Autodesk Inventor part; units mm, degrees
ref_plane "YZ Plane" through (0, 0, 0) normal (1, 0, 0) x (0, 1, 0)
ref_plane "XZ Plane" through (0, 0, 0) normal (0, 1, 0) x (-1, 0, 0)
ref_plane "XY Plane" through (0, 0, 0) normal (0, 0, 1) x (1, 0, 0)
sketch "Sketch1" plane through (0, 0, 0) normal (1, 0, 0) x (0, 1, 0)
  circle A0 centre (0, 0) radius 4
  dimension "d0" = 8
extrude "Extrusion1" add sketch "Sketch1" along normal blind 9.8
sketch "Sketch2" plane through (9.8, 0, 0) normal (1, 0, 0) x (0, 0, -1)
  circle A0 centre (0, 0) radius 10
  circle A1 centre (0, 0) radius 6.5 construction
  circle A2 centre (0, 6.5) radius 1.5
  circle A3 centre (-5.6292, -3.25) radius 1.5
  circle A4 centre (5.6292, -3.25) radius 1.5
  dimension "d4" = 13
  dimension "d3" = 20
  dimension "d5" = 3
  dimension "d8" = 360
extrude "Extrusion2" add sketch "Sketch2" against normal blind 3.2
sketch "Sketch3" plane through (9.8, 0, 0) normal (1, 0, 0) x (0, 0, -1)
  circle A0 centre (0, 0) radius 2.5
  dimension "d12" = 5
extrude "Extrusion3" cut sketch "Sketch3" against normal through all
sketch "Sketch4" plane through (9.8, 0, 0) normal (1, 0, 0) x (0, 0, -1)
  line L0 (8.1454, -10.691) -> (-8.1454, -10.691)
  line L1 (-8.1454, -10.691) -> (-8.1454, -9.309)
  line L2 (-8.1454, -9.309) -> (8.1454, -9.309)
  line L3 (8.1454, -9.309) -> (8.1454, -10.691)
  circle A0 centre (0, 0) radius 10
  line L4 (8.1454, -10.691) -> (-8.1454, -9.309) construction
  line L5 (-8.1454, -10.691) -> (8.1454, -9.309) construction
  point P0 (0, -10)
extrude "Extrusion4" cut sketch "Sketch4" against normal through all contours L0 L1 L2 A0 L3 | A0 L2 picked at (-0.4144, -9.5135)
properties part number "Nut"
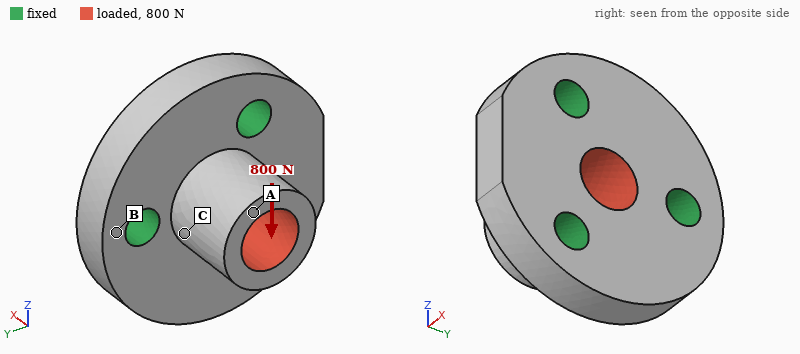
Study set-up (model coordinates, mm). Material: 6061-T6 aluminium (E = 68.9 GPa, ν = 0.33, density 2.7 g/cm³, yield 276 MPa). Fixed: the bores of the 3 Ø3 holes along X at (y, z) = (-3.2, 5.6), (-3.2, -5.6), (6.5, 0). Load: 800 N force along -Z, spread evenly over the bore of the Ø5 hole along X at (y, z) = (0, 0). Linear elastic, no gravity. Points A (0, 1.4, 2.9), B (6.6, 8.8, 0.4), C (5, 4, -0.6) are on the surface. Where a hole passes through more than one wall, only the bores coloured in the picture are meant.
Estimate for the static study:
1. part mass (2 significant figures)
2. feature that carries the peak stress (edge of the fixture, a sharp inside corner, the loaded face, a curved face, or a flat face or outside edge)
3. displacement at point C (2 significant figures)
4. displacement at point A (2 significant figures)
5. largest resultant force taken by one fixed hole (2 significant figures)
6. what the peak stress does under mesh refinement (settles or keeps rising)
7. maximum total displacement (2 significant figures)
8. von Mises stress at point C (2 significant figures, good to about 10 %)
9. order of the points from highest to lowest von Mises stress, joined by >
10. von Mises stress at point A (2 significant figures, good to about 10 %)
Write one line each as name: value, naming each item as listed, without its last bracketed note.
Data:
part mass: 2.9 g
feature that carries the peak stress: a sharp inside corner
displacement at point C: 3.6 µm
displacement at point A: 10 µm
largest resultant force taken by one fixed hole: 360 N
what the peak stress does under mesh refinement: keeps rising
maximum total displacement: 10 µm
von Mises stress at point C: 26 MPa
order of the points from highest to lowest von Mises stress, joined by >: C > A > B
von Mises stress at point A: 16 MPa
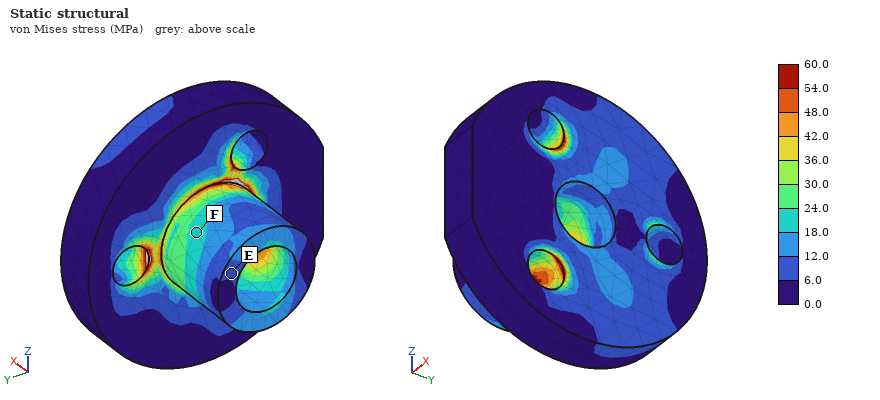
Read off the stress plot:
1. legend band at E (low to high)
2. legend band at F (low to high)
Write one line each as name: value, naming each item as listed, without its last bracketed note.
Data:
legend band at E: 6.0 to 12.0 MPa
legend band at F: 18.0 to 24.0 MPa
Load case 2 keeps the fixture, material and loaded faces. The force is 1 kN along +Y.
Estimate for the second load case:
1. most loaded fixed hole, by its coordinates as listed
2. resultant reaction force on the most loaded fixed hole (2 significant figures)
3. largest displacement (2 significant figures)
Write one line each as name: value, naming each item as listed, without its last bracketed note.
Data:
most loaded fixed hole, by its coordinates as listed: (6.5, 0)
resultant reaction force on the most loaded fixed hole: 480 N
largest displacement: 13 µm
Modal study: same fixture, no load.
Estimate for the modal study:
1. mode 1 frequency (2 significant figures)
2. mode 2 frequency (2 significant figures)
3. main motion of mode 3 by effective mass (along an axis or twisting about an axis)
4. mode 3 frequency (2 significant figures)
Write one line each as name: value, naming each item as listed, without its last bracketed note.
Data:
mode 1 frequency: 54 kHz
mode 2 frequency: 55 kHz
main motion of mode 3 by effective mass: along X
mode 3 frequency: 66 kHz
